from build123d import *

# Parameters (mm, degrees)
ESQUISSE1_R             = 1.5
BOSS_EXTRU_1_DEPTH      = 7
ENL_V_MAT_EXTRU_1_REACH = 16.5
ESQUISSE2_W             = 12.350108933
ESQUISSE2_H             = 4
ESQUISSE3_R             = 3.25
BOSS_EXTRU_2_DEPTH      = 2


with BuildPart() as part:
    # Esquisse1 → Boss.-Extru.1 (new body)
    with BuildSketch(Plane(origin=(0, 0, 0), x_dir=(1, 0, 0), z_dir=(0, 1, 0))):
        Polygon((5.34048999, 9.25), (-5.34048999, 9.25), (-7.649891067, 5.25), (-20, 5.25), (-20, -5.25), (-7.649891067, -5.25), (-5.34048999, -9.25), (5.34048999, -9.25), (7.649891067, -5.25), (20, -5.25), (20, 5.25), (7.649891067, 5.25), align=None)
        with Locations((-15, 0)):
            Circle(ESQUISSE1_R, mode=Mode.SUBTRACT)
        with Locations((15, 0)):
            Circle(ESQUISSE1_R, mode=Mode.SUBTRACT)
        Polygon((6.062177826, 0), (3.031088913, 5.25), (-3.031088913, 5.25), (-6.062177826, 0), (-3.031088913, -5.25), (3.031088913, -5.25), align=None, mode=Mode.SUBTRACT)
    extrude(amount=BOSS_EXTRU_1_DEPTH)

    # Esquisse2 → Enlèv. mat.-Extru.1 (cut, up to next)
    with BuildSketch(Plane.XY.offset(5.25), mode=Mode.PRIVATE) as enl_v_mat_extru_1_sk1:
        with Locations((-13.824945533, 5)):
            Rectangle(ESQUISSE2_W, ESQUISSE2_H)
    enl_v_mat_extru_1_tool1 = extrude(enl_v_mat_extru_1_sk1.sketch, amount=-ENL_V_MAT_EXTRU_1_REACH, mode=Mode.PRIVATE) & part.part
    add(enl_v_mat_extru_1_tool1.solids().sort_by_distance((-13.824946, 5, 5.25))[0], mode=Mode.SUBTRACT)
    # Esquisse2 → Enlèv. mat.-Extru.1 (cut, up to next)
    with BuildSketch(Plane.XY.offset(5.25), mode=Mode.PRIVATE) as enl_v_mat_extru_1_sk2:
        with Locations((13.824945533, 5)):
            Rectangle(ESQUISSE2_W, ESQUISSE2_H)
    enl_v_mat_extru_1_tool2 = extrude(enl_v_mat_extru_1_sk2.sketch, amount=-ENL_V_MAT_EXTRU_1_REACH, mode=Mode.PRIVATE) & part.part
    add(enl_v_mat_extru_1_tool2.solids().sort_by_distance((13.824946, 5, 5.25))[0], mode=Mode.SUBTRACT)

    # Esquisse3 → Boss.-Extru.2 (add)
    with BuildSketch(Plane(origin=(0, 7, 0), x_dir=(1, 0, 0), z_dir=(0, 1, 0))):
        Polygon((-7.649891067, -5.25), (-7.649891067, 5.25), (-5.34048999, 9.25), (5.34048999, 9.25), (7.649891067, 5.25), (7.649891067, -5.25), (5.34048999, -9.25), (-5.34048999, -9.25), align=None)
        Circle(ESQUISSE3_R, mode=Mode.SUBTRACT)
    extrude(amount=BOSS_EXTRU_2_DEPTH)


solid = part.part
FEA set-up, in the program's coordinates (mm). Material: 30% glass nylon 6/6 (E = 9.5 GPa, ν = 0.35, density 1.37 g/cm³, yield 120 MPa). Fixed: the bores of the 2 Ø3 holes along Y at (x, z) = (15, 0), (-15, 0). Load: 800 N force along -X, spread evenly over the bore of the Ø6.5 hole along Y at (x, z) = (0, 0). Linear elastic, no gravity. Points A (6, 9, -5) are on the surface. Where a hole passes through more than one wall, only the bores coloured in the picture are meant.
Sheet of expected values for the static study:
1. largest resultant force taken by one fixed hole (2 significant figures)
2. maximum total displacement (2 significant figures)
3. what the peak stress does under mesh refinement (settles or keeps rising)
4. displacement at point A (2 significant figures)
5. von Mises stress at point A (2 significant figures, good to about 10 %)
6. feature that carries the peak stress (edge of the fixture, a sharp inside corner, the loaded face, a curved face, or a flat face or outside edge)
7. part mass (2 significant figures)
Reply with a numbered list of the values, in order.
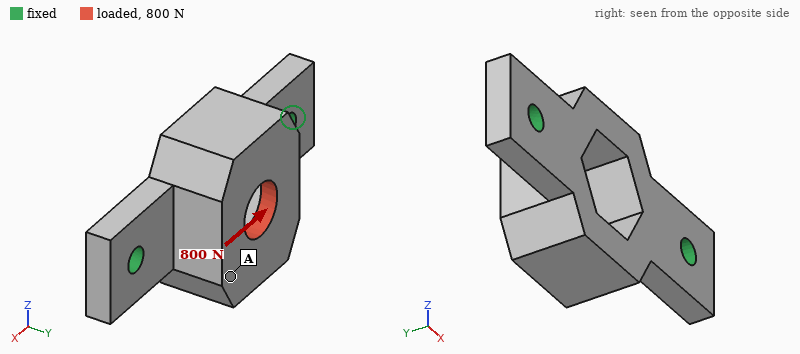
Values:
1. 460 N
2. 99 µm
3. keeps rising
4. 85 µm
5. 14 MPa
6. edge of the fixture
7. 3.3 g
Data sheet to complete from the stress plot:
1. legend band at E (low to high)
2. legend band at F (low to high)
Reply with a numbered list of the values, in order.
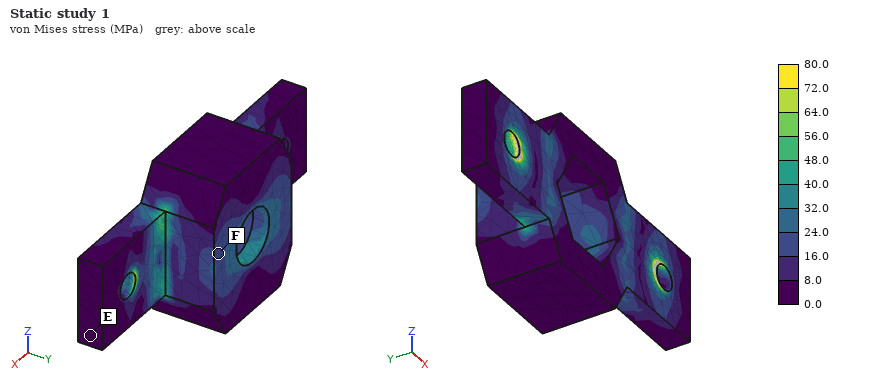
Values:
1. 0.0 to 8.0 MPa
2. 16.0 to 24.0 MPa
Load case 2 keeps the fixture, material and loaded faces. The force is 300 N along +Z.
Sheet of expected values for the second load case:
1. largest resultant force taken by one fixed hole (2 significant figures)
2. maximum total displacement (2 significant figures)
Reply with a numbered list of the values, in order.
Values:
1. 150 N
2. 0.29 mm
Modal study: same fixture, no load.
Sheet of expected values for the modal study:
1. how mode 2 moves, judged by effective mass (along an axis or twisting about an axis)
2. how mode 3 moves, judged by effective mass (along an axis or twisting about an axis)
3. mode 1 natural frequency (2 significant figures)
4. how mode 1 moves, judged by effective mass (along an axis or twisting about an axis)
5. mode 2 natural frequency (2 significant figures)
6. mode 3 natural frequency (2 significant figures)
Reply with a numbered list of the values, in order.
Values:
1. along Y
2. along X
3. 4300 Hz
4. along Z
5. 7700 Hz
6. 13 kHz
